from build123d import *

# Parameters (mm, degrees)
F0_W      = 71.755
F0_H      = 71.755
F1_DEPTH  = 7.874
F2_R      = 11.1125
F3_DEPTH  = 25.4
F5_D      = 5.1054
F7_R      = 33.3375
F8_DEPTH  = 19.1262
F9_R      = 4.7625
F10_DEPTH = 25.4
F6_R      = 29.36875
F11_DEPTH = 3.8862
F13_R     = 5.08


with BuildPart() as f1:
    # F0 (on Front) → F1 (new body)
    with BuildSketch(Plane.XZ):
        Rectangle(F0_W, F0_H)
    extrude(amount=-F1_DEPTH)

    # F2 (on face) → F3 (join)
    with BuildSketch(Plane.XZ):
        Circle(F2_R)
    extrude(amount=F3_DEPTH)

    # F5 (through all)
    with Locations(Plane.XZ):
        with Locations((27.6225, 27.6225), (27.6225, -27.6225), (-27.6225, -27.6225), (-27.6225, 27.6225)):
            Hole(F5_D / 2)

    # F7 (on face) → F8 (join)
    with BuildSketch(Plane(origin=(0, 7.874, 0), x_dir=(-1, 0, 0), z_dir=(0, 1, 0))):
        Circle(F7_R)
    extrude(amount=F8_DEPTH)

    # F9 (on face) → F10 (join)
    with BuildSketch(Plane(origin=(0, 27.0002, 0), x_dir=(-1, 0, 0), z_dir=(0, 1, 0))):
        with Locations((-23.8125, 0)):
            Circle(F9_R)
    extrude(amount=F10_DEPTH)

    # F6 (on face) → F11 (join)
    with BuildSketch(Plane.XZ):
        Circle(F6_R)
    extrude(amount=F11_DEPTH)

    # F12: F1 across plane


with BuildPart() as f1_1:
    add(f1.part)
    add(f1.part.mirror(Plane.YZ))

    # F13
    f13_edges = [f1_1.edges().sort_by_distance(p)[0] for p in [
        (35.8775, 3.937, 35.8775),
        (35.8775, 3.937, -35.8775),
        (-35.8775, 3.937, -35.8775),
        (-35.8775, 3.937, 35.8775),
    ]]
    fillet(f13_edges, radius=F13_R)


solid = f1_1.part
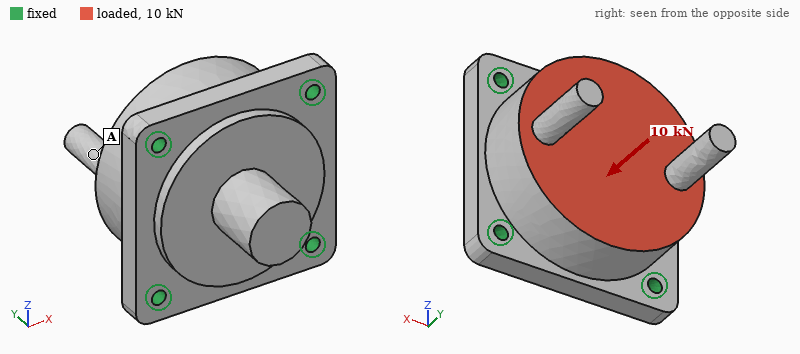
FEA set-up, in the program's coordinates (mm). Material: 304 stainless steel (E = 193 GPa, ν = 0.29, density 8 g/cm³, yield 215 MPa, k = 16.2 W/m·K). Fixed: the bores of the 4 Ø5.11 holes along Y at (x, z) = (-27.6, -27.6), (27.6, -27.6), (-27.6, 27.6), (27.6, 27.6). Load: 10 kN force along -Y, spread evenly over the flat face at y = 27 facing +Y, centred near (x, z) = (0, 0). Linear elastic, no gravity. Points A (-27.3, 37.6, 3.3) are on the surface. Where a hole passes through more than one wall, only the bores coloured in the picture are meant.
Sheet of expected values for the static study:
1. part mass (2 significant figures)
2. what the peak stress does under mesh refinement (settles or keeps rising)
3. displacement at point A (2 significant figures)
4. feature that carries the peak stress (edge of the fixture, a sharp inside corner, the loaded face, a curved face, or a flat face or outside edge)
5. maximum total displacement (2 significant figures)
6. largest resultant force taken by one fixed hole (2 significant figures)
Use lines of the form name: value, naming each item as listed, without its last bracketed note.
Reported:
part mass: 1.0 kg
what the peak stress does under mesh refinement: keeps rising
displacement at point A: 3.8 µm
feature that carries the peak stress: edge of the fixture
maximum total displacement: 4.2 µm
largest resultant force taken by one fixed hole: 2.6 kN
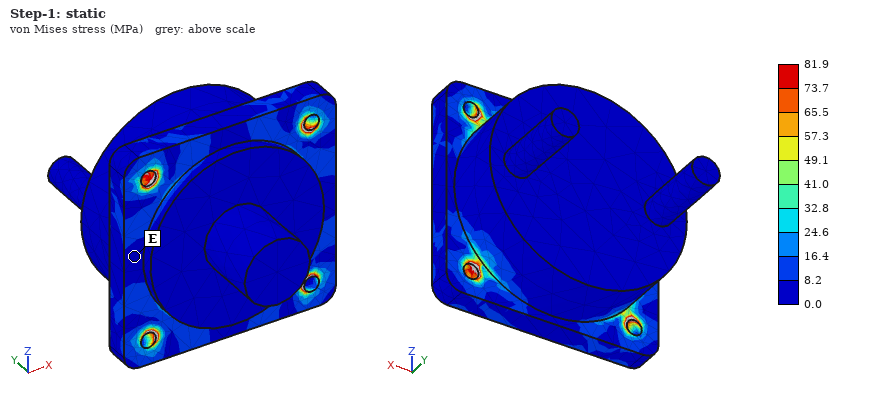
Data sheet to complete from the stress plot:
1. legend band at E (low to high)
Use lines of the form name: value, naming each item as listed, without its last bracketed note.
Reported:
legend band at E: 0.0 to 8.2 MPa
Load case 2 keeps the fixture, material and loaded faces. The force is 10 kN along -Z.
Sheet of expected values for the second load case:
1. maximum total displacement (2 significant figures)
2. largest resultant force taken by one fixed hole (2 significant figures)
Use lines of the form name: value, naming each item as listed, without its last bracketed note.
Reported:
maximum total displacement: 7.2 µm
largest resultant force taken by one fixed hole: 3.5 kN
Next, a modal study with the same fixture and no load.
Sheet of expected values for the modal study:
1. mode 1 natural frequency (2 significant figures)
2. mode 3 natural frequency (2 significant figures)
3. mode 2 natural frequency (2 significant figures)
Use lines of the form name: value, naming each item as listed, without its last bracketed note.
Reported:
mode 1 natural frequency: 7600 Hz
mode 3 natural frequency: 8000 Hz
mode 2 natural frequency: 7700 Hz
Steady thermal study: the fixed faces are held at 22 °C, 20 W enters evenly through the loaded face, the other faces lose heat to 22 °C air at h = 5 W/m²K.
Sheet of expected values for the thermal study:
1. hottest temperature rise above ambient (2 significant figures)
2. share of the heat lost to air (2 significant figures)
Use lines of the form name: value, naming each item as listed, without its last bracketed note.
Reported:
hottest temperature rise above ambient: 26 K
share of the heat lost to air: 6.7 %
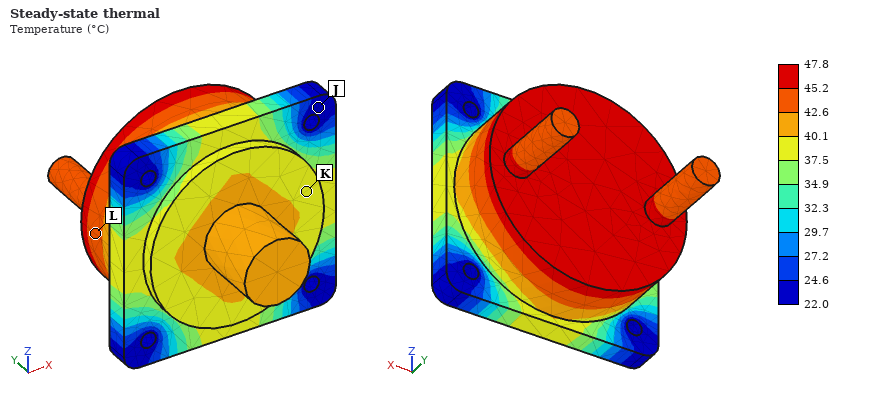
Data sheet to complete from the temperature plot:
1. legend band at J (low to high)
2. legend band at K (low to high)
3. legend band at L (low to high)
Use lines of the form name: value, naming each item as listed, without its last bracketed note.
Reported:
legend band at J: 22.0 to 24.6 °C
legend band at K: 37.5 to 40.1 °C
legend band at L: 42.6 to 45.2 °C
